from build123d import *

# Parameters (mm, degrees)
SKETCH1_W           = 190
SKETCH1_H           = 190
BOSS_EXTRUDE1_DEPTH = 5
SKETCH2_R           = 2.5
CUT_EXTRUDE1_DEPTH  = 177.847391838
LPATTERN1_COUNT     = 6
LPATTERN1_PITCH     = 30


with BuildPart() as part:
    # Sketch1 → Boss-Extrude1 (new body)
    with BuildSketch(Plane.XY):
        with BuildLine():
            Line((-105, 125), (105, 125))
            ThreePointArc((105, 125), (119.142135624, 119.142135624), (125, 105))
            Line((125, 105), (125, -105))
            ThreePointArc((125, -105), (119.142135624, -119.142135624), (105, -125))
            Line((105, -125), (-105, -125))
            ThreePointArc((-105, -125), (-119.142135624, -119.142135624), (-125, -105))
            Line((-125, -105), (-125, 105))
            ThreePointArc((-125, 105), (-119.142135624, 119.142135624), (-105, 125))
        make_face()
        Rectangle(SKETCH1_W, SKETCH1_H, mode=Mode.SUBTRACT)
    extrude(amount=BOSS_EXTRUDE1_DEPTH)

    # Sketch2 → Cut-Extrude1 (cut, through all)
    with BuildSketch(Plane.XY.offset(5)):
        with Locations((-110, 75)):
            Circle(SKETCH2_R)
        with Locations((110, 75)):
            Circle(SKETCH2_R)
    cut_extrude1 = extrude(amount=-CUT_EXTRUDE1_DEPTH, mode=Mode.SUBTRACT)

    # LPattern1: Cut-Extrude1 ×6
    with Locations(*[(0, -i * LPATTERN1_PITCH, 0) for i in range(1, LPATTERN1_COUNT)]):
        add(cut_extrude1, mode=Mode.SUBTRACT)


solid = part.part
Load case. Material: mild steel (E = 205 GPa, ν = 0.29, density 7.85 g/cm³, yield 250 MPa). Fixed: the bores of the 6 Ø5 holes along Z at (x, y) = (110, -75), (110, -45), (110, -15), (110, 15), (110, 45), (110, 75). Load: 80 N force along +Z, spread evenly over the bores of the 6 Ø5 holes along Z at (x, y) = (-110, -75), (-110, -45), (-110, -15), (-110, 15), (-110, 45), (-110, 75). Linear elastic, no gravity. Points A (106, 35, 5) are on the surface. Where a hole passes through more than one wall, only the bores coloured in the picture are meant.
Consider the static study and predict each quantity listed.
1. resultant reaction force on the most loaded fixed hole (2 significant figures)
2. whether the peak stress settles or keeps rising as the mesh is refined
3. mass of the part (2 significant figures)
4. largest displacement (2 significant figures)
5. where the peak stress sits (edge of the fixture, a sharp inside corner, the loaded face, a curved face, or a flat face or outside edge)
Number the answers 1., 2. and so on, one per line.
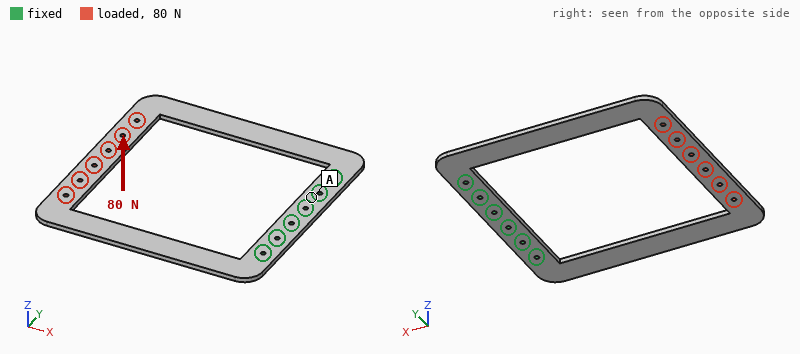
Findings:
1. 49 N
2. keeps rising
3. 1.0 kg
4. 3.0 mm
5. edge of the fixture
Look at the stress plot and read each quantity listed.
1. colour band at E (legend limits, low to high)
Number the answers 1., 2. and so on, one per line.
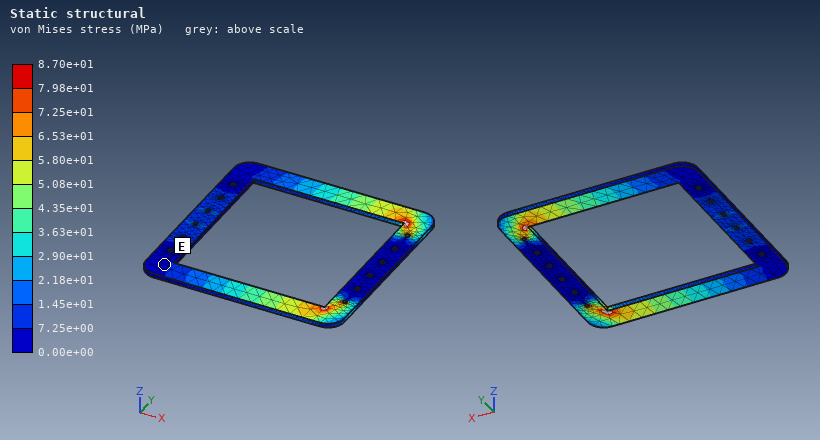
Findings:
1. 0.00e+00 to 7.25e+00 MPa
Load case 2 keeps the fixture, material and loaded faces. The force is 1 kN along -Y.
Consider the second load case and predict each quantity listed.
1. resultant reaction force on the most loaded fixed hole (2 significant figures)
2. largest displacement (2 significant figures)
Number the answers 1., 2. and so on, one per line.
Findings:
1. 2.3 kN
2. 0.47 mm
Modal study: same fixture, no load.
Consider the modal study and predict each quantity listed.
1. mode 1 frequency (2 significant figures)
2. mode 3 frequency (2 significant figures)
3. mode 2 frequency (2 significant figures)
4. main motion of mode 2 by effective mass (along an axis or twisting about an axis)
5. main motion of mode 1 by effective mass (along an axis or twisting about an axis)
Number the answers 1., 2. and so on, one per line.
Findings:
1. 45 Hz
2. 300 Hz
3. 100 Hz
4. twisting about X
5. along Z
